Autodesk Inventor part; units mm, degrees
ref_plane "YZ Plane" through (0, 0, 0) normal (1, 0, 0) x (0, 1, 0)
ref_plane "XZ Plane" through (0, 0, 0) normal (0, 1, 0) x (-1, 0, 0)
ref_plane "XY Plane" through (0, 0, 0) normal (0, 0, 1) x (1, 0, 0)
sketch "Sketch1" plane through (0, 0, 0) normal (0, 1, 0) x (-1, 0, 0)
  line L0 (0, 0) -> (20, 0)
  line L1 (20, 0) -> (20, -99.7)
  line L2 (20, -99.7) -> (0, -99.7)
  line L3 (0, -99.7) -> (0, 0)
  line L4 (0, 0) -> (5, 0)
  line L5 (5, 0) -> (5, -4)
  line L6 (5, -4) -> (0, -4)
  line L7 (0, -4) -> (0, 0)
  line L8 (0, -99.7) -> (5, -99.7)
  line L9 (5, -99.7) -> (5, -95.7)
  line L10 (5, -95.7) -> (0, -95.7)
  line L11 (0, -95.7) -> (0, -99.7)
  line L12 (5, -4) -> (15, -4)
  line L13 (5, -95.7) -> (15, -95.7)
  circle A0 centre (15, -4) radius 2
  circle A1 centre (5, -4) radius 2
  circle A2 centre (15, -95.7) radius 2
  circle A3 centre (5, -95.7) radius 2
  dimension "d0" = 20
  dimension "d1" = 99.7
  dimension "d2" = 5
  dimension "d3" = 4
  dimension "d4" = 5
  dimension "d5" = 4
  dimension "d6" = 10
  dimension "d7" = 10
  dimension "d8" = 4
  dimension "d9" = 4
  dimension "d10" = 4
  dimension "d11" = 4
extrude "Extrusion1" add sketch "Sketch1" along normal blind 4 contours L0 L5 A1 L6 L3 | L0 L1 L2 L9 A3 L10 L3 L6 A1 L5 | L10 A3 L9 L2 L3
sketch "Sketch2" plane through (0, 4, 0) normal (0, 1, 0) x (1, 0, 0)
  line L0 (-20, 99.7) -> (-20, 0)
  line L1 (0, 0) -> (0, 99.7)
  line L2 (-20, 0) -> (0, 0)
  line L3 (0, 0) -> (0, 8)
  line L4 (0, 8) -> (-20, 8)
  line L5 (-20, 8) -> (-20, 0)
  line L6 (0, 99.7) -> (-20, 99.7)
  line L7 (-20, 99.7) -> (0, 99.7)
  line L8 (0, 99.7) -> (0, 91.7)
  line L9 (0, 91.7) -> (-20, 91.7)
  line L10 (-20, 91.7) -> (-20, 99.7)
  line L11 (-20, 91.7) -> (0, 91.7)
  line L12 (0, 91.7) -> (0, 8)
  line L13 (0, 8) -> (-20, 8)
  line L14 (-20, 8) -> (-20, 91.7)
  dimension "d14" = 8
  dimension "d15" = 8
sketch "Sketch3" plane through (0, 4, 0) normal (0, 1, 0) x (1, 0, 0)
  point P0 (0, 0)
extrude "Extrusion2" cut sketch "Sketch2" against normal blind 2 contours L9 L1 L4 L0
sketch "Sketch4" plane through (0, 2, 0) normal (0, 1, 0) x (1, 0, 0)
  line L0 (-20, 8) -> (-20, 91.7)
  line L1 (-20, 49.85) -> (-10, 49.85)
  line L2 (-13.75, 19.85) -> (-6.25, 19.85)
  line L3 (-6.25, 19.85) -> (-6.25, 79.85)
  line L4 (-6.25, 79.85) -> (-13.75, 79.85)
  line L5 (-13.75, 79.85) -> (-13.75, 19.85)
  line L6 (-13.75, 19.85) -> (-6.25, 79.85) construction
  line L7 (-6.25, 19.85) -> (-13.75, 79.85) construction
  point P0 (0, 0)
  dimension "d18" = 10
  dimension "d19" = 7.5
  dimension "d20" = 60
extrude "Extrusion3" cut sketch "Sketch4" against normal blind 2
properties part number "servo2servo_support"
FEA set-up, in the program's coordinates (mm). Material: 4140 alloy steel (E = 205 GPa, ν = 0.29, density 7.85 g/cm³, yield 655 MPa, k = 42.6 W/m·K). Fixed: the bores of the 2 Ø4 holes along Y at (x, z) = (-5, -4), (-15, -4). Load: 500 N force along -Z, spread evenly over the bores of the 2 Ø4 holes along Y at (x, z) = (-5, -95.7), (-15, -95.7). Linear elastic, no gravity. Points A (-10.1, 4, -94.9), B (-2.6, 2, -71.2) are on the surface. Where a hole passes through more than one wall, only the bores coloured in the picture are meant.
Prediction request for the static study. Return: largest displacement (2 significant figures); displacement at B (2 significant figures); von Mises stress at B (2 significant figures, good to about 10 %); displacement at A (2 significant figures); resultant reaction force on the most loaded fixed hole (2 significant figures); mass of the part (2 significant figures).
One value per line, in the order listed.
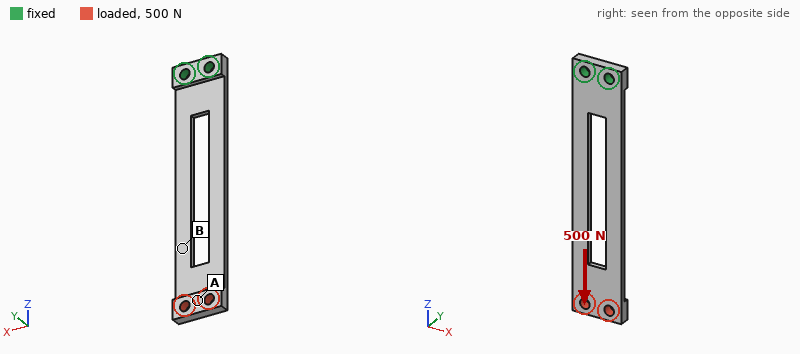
1.1 mm
0.53 mm
80 MPa
1.0 mm
250 N
28 g
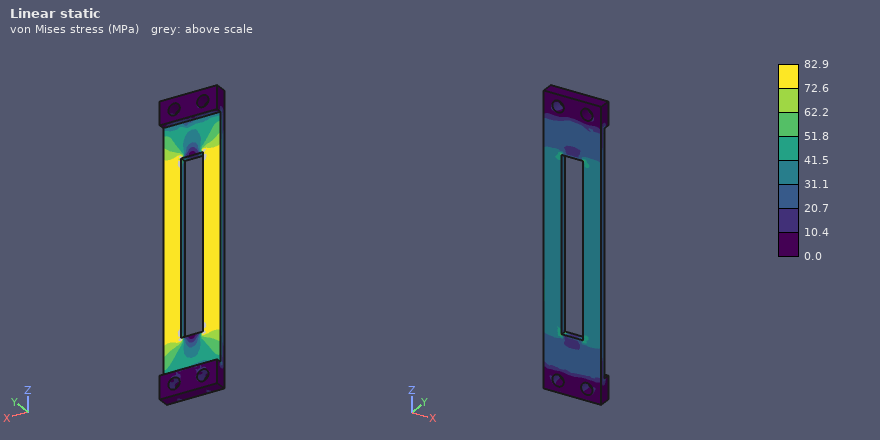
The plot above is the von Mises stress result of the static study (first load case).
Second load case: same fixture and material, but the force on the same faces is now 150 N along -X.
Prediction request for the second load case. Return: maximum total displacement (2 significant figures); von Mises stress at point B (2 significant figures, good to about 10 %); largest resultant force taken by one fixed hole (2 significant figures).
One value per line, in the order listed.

0.38 mm
41 MPa
1.1 kN
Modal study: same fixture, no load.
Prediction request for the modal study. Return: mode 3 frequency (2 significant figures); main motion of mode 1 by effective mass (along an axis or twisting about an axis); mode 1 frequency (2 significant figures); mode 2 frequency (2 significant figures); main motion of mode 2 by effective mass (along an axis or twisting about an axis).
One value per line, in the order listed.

1100 Hz
along Y
160 Hz
990 Hz
along X
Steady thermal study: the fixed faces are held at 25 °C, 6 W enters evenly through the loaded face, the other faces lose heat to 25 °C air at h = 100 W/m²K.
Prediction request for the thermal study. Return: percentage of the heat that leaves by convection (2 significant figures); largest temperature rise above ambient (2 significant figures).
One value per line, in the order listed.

99 %
56 K
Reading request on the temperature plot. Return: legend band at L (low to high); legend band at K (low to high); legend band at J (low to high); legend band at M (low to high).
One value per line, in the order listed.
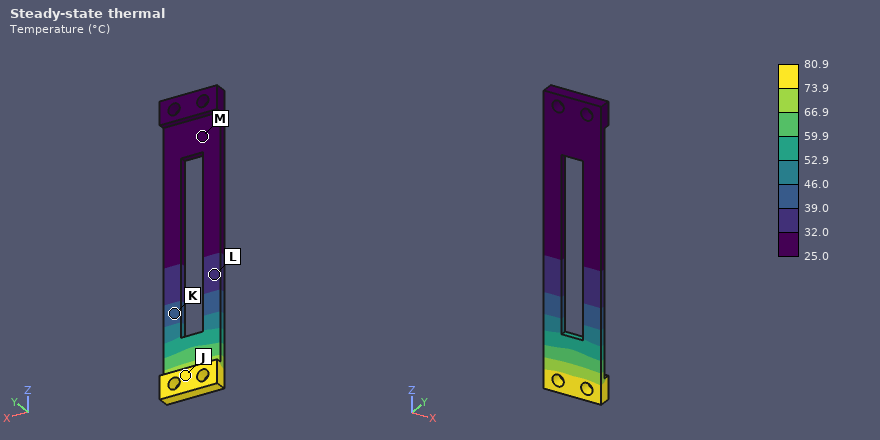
32.0 to 39.0 °C
39.0 to 46.0 °C
73.9 to 80.9 °C
25.0 to 32.0 °C
